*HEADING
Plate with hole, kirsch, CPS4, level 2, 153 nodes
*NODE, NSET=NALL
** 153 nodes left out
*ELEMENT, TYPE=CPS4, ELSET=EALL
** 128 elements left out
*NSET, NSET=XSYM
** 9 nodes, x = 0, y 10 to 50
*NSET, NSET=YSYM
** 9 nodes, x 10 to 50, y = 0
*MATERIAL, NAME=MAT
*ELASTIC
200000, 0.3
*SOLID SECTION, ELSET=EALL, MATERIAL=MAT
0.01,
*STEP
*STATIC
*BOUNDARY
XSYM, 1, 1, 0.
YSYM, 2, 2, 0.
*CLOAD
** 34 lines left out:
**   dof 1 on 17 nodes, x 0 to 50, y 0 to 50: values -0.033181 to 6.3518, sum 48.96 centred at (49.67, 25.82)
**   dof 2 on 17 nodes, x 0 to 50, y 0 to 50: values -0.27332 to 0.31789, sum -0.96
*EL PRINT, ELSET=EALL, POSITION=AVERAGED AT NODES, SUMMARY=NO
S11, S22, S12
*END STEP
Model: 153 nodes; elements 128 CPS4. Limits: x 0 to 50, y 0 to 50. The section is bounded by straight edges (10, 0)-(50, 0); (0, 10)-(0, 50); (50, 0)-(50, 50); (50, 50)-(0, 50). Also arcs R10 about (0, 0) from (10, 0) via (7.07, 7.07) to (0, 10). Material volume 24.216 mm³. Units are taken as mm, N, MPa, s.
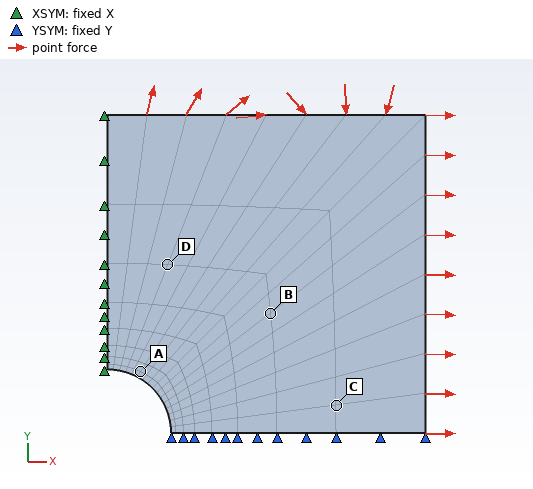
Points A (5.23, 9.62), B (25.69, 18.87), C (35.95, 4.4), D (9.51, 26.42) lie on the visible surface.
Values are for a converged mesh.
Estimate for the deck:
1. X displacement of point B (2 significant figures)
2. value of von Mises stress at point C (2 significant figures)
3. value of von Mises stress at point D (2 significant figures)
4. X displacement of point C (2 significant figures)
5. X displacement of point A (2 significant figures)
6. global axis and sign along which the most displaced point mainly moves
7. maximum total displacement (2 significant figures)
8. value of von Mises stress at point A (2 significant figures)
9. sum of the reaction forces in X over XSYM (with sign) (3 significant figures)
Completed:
0.015 mm
80 MPa
110 MPa
0.021 mm
0.0065 mm
+X
0.028 mm
170 MPa
-49.0 N
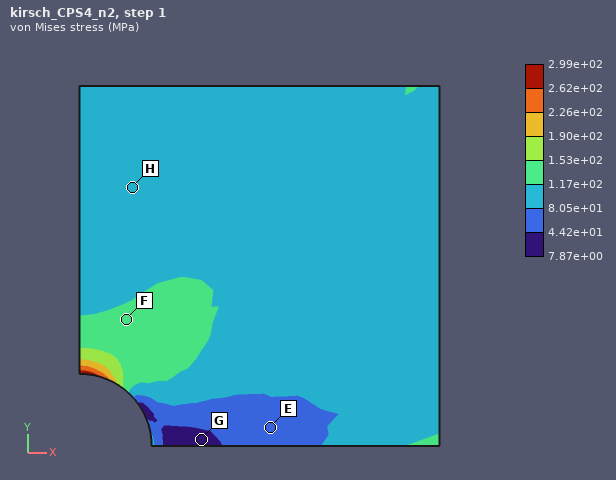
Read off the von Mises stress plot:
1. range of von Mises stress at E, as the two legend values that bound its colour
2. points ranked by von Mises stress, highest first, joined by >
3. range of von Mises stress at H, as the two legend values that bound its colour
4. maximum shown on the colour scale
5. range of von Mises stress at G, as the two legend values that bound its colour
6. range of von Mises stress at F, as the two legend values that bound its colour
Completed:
4.42e+01 to 8.05e+01 MPa
F > H > E > G
8.05e+01 to 1.17e+02 MPa
2.99e+02 MPa
7.87e+00 to 4.42e+01 MPa
1.17e+02 to 1.53e+02 MPa
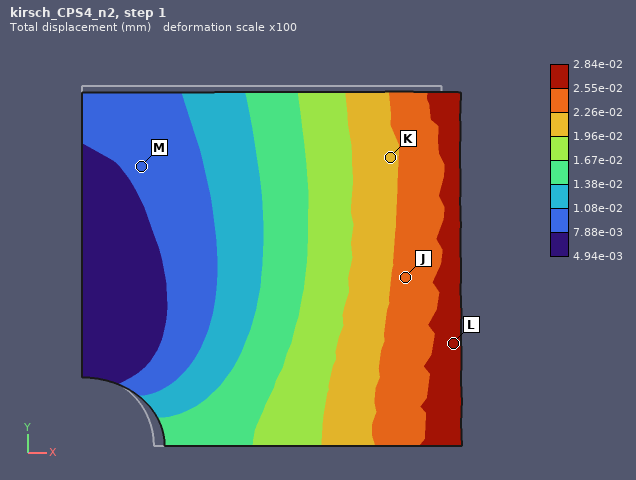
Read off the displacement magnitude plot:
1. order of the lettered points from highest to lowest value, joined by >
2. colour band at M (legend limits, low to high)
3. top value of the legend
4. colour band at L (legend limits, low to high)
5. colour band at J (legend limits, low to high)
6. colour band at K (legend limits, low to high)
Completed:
L > J > K > M
7.88e-03 to 1.08e-02 mm
2.84e-02 mm
2.55e-02 to 2.84e-02 mm
2.26e-02 to 2.55e-02 mm
1.96e-02 to 2.26e-02 mm
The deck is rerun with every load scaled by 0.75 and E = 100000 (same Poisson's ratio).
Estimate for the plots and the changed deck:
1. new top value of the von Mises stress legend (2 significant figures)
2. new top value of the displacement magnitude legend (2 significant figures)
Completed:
220 MPa
0.043 mm
